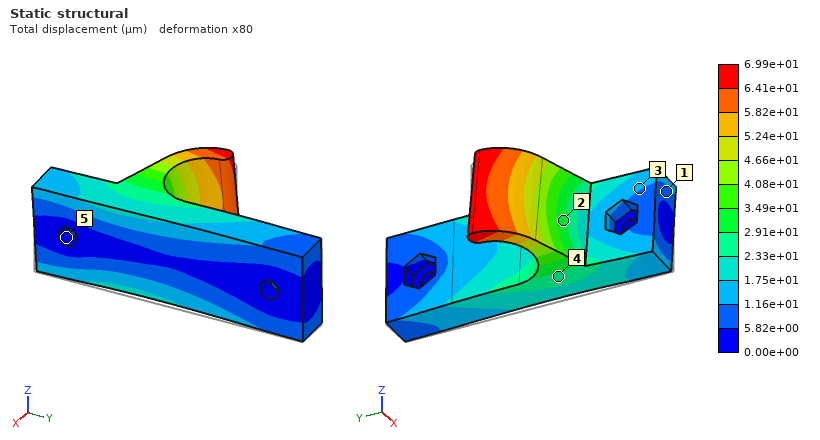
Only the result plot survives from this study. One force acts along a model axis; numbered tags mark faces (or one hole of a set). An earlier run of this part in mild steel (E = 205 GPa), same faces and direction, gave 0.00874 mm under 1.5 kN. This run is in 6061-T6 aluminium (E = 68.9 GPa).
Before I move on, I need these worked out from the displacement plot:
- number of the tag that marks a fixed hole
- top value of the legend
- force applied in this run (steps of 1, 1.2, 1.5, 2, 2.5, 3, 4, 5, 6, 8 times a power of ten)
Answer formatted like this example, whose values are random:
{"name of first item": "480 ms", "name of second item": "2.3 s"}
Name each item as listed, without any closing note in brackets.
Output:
{"number of the tag that marks a fixed hole": "5", "top value of the legend": "6.99e+01 µm", "force applied in this run": "4 kN"}
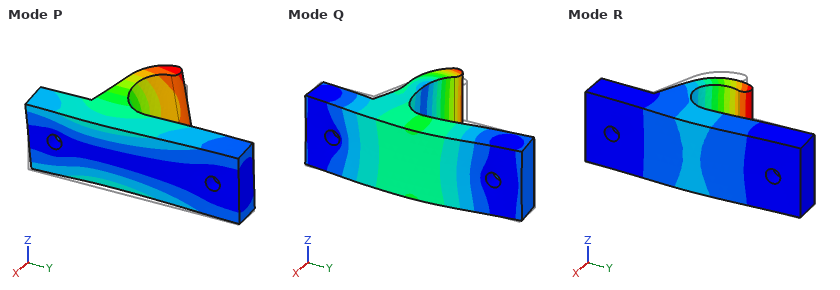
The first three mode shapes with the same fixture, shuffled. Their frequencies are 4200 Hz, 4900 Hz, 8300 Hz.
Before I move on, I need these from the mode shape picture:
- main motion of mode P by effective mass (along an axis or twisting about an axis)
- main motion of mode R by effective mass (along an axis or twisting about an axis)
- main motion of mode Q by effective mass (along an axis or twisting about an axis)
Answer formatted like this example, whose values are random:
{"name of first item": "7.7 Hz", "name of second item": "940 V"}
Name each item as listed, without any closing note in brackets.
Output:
{"main motion of mode P by effective mass": "along Z", "main motion of mode R by effective mass": "along X", "main motion of mode Q by effective mass": "along X"}
